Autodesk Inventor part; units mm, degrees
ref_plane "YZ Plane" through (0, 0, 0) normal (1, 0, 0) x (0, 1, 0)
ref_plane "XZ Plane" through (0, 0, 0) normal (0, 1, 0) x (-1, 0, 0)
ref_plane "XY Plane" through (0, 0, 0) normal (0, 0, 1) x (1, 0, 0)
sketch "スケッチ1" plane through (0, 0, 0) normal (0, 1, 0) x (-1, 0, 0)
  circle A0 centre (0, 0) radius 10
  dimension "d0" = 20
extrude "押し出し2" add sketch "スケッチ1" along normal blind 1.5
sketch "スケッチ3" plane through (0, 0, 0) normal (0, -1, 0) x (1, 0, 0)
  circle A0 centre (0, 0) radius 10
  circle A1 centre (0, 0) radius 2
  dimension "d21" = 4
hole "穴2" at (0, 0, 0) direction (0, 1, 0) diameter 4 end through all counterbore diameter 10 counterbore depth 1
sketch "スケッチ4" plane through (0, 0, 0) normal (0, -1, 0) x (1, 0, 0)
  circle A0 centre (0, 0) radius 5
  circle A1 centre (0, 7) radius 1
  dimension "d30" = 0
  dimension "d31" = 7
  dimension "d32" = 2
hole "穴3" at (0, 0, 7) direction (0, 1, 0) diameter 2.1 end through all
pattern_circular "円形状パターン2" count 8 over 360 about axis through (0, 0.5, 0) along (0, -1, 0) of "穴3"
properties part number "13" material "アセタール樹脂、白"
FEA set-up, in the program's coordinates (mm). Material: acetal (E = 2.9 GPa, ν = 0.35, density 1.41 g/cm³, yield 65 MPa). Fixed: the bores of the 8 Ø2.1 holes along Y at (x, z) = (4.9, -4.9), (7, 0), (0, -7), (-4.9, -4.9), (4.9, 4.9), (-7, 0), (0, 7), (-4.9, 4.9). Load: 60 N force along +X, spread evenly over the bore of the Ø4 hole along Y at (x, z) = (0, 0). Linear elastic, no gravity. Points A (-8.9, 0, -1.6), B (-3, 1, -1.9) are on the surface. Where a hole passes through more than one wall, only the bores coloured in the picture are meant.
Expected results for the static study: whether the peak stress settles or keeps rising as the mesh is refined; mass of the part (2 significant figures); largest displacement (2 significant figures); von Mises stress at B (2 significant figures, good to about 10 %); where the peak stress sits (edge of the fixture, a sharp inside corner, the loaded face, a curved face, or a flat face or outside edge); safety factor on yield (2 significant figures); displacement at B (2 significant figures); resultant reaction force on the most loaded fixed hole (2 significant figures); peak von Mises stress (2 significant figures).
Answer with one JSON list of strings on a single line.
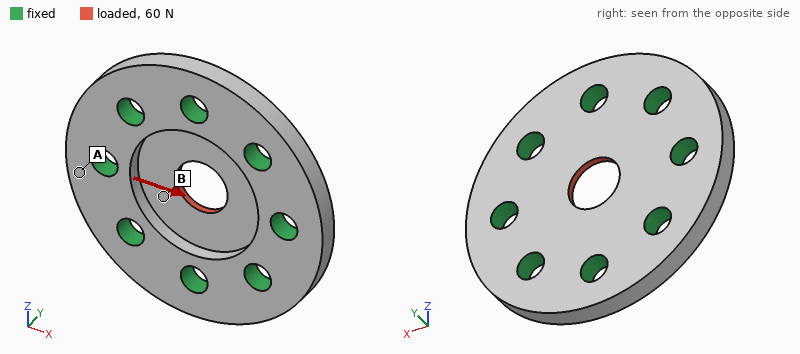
["settles", "0.49 g", "12 µm", "7.4 MPa", "the loaded face", "3.9", "6.4 µm", "13 N", "17 MPa"]
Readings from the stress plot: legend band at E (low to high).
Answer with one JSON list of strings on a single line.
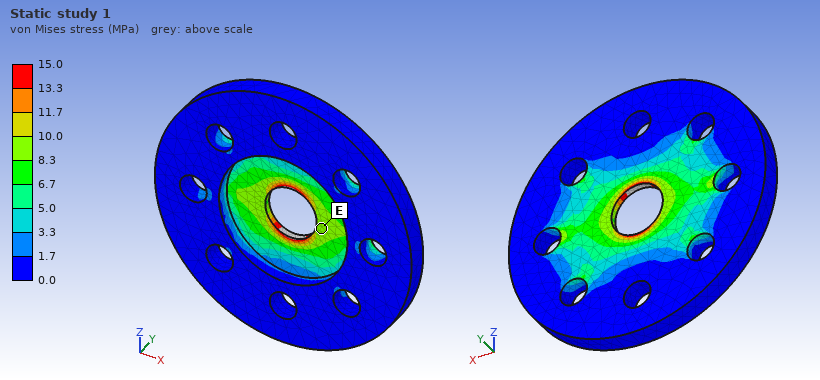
["8.3 to 10.0 MPa"]
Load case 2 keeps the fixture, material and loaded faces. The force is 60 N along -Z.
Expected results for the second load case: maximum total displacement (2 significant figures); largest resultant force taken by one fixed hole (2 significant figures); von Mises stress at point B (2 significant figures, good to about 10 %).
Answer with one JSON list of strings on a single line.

["12 µm", "13 N", "6.4 MPa"]
